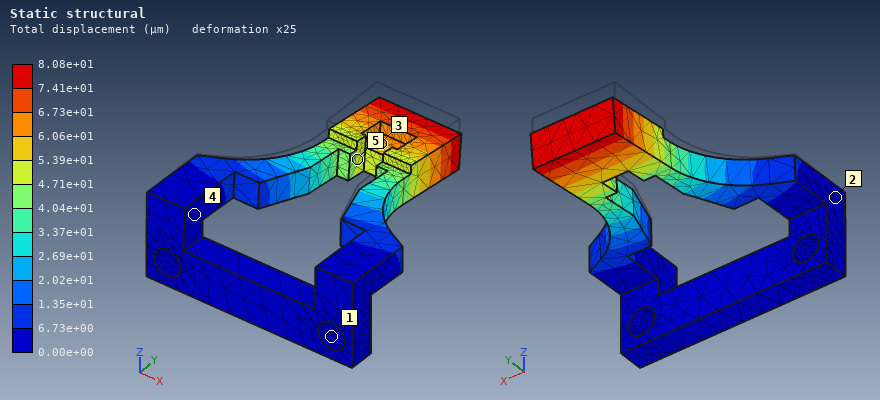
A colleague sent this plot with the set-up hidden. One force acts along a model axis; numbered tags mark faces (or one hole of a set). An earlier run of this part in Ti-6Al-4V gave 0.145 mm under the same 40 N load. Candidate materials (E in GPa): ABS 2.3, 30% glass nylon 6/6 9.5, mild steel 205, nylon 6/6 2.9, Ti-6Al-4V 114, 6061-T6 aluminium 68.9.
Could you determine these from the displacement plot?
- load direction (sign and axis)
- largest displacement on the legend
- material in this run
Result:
-Z
8.08e+01 µm
mild steel
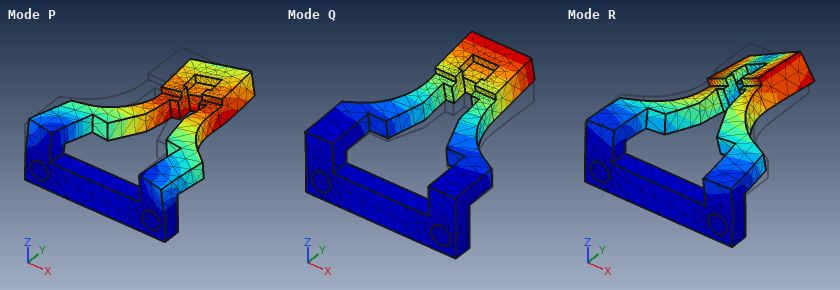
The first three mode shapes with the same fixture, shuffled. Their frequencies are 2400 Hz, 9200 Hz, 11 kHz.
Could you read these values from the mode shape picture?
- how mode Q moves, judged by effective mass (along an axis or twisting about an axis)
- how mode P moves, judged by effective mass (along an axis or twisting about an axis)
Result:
along Z
along X
